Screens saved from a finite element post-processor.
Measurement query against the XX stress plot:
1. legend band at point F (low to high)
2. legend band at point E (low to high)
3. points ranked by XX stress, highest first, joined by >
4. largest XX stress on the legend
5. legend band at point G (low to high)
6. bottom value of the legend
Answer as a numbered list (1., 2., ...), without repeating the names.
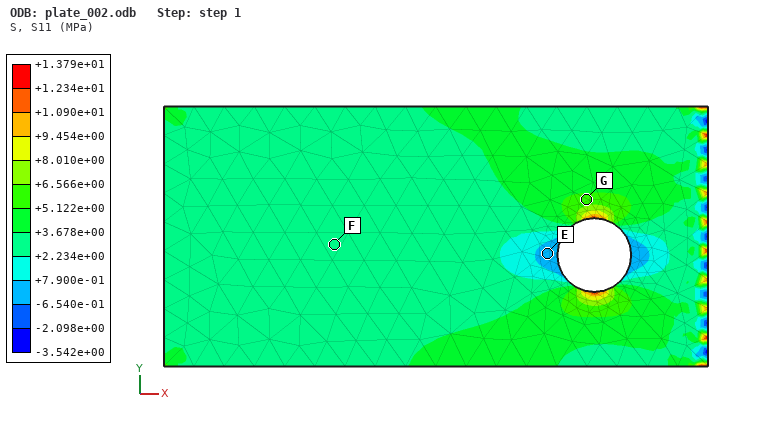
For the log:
1. +2.234e+00 to +3.678e+00 MPa
2. -6.540e-01 to +7.900e-01 MPa
3. G > F > E
4. +1.379e+01 MPa
5. +5.122e+00 to +6.566e+00 MPa
6. -3.542e+00 MPa
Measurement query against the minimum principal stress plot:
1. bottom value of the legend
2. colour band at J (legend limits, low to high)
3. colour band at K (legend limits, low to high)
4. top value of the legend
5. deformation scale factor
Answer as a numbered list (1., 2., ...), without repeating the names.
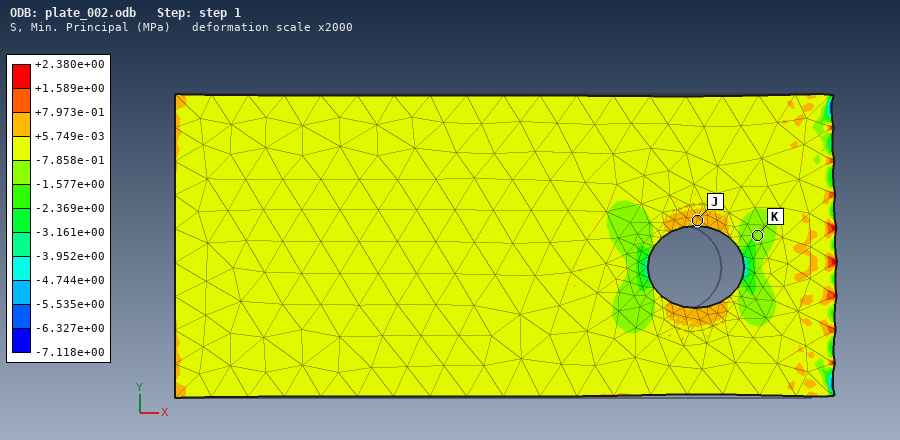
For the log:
1. -7.118e+00 MPa
2. +5.749e-03 to +7.973e-01 MPa
3. -1.577e+00 to -7.858e-01 MPa
4. +2.380e+00 MPa
5. 2000
